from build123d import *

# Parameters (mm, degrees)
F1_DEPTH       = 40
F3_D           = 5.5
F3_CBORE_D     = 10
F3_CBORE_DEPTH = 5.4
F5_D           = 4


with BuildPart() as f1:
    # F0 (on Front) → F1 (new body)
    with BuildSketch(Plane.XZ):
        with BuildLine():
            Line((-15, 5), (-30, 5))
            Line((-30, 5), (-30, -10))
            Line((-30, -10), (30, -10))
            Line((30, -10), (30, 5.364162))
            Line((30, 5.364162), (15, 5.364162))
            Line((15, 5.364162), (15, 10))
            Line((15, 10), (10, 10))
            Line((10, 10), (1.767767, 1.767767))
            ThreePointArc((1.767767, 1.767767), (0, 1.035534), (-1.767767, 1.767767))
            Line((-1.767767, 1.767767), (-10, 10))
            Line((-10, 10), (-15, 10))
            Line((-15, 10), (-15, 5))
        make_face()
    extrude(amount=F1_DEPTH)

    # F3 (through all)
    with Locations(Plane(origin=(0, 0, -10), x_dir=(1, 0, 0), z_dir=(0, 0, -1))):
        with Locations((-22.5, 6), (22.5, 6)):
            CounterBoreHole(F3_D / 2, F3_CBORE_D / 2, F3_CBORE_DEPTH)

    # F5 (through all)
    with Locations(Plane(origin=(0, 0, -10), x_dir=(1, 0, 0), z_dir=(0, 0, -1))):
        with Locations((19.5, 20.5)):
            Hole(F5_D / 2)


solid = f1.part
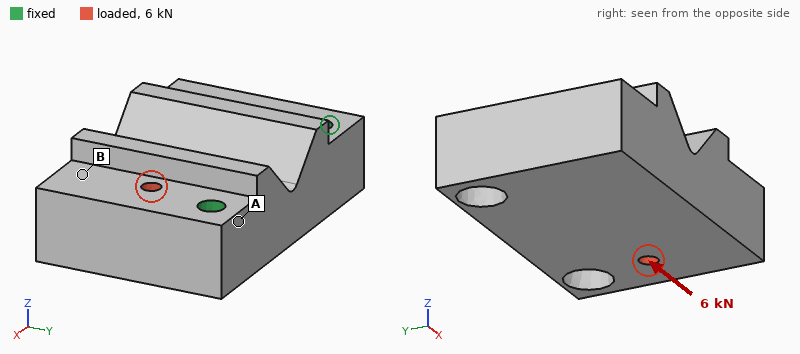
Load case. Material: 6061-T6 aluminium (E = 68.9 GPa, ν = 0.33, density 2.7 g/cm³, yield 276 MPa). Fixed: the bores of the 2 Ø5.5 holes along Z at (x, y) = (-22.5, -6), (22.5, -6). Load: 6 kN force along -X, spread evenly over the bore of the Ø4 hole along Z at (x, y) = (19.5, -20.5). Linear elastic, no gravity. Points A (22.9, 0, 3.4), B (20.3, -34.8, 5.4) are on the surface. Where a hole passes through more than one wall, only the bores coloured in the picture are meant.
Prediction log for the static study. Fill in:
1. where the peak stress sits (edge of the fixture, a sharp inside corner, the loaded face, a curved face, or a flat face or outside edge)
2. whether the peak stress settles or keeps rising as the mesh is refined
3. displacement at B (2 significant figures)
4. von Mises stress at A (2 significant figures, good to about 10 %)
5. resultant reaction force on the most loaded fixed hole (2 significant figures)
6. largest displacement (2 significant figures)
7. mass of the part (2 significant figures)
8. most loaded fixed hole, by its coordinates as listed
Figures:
edge of the fixture
keeps rising
9.2 µm
13 MPa
4.1 kN
11 µm
99 g
(22.5, -6)
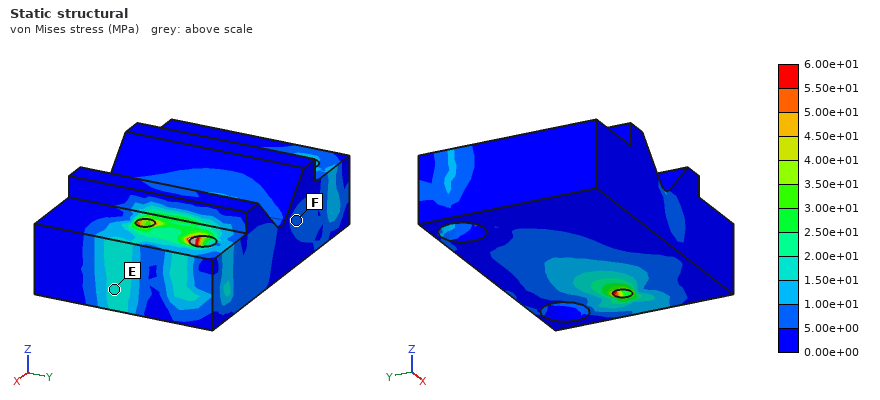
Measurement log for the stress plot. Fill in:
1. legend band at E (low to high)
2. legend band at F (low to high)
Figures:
1.50e+01 to 2.00e+01 MPa
5.00e+00 to 1.00e+01 MPa
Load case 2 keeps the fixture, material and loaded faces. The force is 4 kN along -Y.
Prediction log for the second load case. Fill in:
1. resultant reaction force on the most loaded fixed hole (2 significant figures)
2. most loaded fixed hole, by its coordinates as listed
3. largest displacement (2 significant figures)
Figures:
3.7 kN
(22.5, -6)
12 µm
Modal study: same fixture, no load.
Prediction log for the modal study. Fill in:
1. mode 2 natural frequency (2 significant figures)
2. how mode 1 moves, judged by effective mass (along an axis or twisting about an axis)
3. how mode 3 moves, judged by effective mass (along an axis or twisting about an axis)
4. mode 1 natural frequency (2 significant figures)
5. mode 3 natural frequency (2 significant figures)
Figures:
11 kHz
along Z
along X
5100 Hz
15 kHz
